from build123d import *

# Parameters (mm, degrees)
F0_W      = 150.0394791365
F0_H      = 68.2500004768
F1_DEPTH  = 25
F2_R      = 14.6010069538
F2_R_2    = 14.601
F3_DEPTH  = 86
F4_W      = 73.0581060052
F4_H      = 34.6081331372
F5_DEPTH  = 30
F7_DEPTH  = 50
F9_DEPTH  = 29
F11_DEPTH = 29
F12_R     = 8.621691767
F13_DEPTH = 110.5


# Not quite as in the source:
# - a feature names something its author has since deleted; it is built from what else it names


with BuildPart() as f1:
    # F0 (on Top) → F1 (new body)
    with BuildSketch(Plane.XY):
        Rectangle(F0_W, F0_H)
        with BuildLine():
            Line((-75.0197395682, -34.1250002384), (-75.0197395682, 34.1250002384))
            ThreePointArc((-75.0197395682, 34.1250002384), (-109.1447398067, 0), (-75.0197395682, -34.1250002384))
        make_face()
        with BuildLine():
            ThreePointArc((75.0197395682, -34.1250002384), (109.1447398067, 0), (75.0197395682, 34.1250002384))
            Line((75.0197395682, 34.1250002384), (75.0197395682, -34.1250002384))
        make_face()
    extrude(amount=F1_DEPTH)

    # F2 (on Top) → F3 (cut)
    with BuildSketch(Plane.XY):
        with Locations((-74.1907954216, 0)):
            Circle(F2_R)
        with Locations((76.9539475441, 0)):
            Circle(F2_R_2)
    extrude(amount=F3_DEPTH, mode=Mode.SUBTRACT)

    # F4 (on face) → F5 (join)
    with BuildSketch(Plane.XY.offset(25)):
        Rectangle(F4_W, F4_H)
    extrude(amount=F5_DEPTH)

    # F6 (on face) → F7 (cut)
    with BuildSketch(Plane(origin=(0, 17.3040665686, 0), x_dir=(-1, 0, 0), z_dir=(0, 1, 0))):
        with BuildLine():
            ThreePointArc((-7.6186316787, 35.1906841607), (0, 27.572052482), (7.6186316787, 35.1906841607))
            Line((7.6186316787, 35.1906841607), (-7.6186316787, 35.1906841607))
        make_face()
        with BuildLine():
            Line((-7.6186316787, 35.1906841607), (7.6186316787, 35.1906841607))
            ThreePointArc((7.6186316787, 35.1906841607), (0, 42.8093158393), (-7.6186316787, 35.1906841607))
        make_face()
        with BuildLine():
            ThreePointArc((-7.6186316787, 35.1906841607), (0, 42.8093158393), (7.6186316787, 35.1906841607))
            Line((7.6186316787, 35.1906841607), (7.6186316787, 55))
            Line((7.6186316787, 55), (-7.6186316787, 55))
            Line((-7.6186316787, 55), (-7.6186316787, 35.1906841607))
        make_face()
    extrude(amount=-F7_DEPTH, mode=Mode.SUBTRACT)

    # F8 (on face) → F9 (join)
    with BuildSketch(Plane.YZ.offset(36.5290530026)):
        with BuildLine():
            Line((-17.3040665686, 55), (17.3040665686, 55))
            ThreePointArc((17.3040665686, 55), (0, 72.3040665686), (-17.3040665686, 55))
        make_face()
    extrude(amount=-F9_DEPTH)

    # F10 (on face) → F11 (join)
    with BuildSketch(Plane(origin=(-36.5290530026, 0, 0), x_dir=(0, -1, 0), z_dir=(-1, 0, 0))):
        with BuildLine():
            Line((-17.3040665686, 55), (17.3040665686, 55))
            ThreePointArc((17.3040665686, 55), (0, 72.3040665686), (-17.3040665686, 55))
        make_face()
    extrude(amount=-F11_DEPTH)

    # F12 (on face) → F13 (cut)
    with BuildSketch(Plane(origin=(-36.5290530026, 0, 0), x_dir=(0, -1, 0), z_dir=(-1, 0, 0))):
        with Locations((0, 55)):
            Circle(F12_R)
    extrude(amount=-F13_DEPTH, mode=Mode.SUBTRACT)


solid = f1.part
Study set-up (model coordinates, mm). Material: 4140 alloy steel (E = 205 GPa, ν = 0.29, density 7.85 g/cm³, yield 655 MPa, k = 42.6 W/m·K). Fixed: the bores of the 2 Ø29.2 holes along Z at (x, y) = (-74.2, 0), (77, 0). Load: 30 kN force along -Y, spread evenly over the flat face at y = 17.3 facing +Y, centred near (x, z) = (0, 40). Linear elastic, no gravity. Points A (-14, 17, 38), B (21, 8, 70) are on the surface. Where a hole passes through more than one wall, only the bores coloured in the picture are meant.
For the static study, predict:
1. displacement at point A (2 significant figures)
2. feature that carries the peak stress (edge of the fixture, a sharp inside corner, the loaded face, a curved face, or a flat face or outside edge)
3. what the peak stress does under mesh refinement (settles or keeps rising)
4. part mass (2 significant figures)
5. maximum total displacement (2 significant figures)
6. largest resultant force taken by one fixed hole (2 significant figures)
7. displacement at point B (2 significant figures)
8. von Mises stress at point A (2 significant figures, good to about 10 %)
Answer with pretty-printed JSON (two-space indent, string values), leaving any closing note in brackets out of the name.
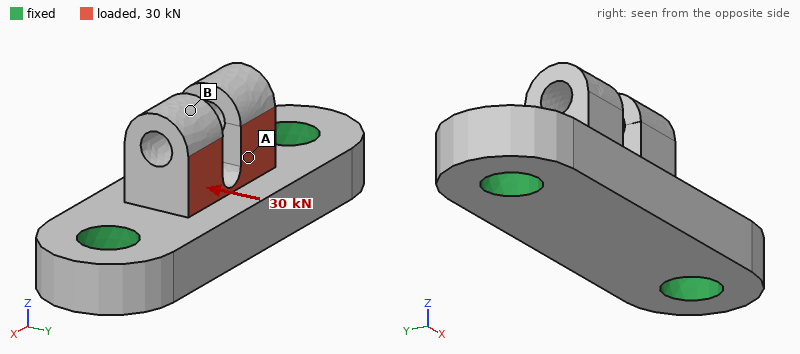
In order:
{
  "displacement at point A": "31 µm",
  "feature that carries the peak stress": "edge of the fixture",
  "what the peak stress does under mesh refinement": "keeps rising",
  "part mass": "3.1 kg",
  "maximum total displacement": "55 µm",
  "largest resultant force taken by one fixed hole": "15 kN",
  "displacement at point B": "54 µm",
  "von Mises stress at point A": "25 MPa"
}
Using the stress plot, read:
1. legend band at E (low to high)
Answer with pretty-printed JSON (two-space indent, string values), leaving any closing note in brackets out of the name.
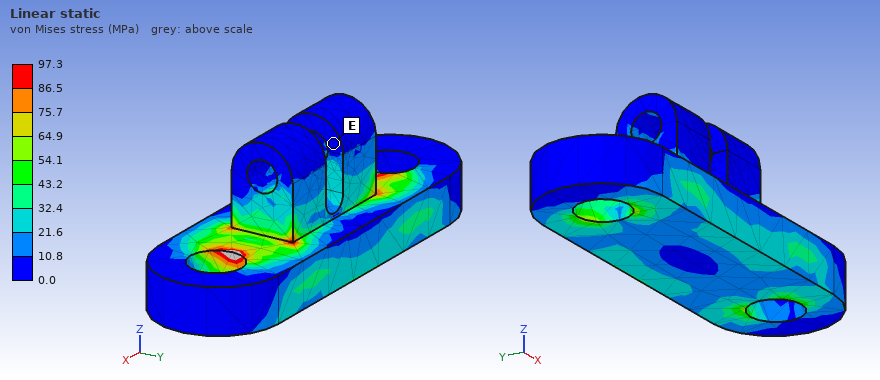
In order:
{
  "legend band at E": "0.0 to 10.8 MPa"
}
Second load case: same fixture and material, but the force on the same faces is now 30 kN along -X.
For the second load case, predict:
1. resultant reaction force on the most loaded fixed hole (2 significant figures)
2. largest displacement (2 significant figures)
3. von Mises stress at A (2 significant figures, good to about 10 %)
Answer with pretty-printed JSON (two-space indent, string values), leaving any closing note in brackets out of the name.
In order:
{
  "resultant reaction force on the most loaded fixed hole": "17 kN",
  "largest displacement": "24 µm",
  "von Mises stress at A": "72 MPa"
}
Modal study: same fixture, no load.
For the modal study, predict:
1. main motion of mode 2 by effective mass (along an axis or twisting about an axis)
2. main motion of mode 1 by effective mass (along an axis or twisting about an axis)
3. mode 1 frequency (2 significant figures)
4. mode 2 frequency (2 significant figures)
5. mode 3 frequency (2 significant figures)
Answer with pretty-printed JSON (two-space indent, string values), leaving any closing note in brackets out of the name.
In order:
{
  "main motion of mode 2 by effective mass": "along Z",
  "main motion of mode 1 by effective mass": "along Y",
  "mode 1 frequency": "4500 Hz",
  "mode 2 frequency": "5000 Hz",
  "mode 3 frequency": "7800 Hz"
}
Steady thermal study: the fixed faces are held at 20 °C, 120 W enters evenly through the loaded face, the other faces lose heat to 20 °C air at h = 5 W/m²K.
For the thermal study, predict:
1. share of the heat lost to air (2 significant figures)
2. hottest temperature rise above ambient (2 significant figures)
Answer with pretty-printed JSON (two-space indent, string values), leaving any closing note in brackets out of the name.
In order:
{
  "share of the heat lost to air": "5.2 %",
  "hottest temperature rise above ambient": "76 K"
}
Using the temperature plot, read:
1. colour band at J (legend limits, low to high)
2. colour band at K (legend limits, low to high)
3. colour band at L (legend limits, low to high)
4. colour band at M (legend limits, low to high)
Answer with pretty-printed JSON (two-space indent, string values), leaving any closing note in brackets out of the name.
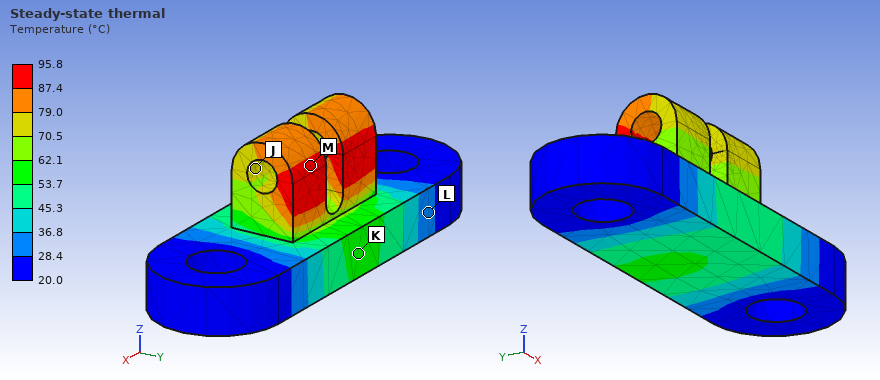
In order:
{
  "colour band at J": "70.5 to 79.0 °C",
  "colour band at K": "53.7 to 62.1 °C",
  "colour band at L": "28.4 to 36.8 °C",
  "colour band at M": "87.4 to 95.8 °C"
}
